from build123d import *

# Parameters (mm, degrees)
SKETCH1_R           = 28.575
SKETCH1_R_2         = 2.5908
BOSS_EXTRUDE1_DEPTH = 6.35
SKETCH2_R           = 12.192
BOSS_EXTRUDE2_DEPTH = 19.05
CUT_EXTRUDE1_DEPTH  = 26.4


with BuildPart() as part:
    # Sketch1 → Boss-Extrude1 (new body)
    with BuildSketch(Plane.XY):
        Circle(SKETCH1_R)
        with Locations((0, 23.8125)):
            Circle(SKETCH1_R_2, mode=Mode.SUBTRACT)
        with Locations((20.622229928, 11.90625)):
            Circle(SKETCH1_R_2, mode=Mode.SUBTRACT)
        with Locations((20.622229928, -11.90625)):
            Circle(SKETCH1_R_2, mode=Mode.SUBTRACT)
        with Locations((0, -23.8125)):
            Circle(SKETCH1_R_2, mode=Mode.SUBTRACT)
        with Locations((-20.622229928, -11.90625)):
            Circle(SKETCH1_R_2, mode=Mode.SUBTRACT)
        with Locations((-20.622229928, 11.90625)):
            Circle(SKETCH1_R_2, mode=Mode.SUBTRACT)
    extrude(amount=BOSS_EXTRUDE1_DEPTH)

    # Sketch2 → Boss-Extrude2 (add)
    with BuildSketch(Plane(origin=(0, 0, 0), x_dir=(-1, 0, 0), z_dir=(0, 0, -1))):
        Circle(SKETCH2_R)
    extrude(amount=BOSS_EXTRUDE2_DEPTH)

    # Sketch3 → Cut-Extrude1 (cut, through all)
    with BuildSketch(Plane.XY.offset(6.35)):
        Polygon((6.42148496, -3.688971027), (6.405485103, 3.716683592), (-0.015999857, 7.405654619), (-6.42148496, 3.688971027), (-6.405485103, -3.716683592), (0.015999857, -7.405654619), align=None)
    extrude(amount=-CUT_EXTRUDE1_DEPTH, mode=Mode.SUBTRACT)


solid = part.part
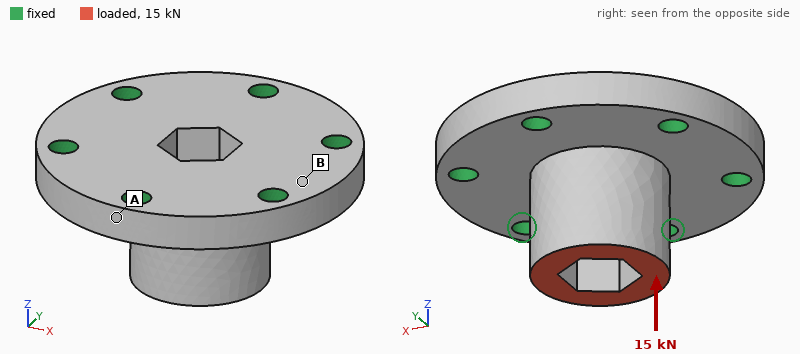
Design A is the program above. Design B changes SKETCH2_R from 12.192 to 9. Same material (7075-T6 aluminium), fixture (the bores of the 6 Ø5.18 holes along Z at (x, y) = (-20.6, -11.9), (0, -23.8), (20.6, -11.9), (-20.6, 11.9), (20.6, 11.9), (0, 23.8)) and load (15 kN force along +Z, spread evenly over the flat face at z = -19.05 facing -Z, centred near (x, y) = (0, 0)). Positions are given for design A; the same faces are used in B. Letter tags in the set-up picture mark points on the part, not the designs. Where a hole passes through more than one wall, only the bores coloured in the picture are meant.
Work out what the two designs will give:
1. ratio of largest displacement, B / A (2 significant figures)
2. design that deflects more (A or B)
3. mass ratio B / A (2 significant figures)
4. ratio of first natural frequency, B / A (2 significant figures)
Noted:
2.1
B
0.81
1.0
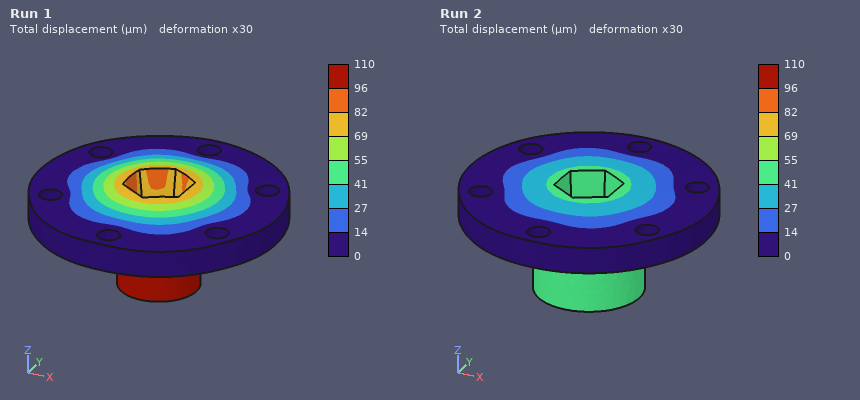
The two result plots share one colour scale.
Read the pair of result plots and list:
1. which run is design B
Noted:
Run 1
